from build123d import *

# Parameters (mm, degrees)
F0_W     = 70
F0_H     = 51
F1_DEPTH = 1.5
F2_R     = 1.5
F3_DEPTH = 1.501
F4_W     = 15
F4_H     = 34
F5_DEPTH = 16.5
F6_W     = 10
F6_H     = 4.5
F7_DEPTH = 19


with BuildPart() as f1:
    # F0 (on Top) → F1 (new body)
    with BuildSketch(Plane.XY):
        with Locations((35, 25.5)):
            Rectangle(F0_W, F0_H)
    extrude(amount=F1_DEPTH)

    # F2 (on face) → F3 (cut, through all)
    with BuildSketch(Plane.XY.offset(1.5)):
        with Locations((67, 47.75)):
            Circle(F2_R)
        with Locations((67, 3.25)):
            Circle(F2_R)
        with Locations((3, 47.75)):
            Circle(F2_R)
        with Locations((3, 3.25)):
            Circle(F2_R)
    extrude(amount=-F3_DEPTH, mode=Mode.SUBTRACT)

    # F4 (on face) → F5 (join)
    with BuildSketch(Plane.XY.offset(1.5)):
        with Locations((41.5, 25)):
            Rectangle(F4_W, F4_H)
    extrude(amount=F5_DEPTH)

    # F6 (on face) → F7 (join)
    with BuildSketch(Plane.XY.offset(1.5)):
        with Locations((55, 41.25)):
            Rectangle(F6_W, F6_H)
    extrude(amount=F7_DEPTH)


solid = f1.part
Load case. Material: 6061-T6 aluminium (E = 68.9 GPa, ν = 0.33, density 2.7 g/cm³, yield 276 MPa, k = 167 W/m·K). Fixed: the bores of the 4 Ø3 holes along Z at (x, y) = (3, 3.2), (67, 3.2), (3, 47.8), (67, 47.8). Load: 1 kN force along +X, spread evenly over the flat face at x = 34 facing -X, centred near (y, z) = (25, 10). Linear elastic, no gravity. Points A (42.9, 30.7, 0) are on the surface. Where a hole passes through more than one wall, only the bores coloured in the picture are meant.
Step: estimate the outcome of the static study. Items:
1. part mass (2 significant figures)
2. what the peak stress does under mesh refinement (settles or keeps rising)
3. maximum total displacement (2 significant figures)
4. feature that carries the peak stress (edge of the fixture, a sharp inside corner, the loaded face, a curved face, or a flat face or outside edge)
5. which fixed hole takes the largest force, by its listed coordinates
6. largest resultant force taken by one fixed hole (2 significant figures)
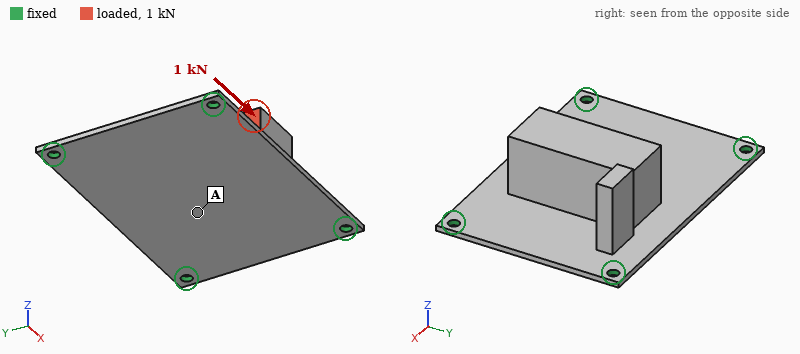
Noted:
39 g
keeps rising
0.47 mm
edge of the fixture
(67, 47.8)
330 N
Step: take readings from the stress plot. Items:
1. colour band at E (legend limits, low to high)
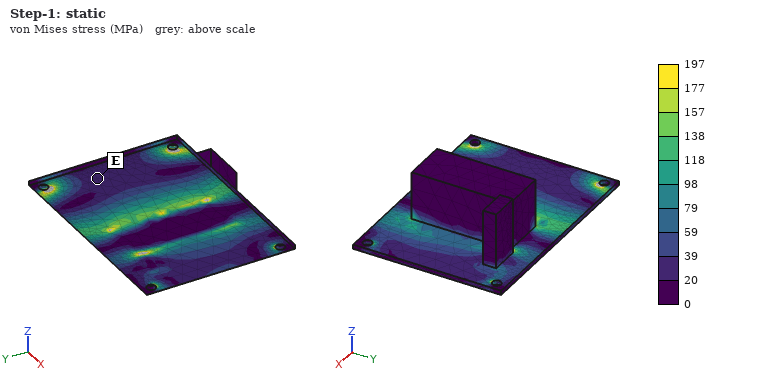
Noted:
20 to 39 MPa
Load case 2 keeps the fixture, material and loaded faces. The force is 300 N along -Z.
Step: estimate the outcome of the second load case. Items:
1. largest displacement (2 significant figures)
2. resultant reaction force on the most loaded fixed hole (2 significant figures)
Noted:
0.46 mm
87 N
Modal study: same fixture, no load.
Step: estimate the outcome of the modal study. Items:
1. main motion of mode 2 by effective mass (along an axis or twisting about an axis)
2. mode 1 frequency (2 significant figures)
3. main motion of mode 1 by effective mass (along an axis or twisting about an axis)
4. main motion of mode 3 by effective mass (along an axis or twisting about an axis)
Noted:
along Y
890 Hz
along Z
along X
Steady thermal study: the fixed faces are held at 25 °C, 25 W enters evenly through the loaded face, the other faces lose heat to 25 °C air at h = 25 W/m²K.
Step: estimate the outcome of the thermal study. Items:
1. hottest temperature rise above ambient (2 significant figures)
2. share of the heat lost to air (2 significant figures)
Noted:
34 K
19 %
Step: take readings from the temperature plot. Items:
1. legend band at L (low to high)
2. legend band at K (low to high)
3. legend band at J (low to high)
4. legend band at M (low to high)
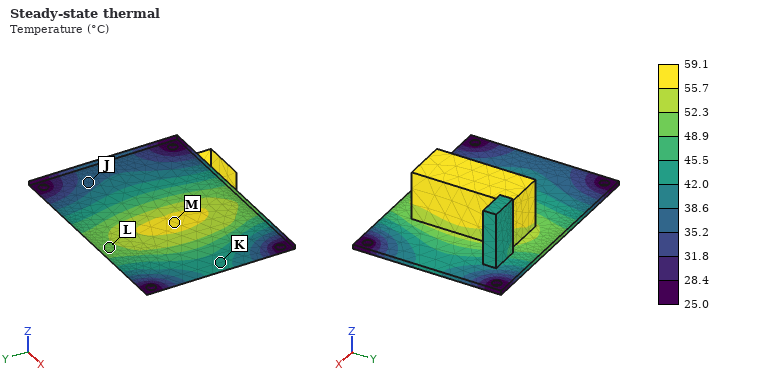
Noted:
48.9 to 52.3 °C
42.0 to 45.5 °C
35.2 to 38.6 °C
55.7 to 59.1 °C
